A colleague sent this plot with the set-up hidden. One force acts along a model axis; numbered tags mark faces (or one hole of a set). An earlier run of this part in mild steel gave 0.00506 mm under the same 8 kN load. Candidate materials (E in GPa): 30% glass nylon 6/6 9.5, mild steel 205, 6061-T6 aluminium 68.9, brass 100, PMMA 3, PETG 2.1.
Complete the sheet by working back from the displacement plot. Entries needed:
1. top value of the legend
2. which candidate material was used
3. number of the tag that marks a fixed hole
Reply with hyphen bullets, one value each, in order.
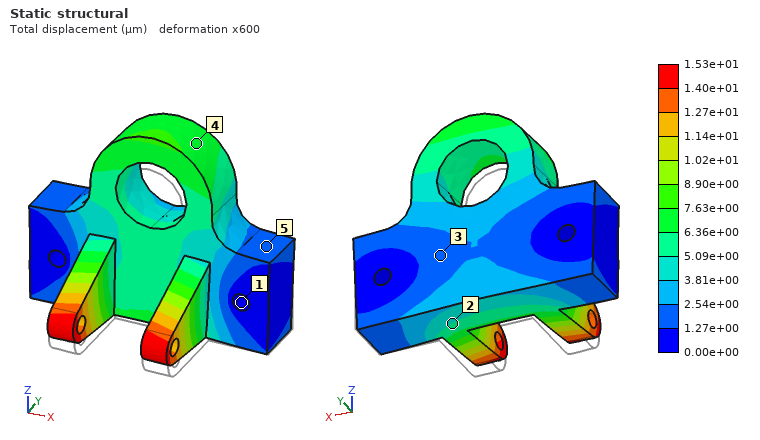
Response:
- 1.53e+01 µm
- 6061-T6 aluminium
- 1
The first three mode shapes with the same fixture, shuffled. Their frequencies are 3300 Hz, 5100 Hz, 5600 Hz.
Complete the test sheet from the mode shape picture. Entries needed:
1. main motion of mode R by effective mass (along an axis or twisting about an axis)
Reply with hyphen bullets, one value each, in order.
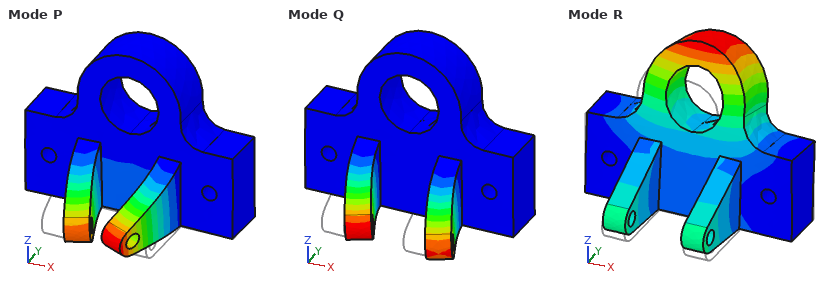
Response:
- along Y
